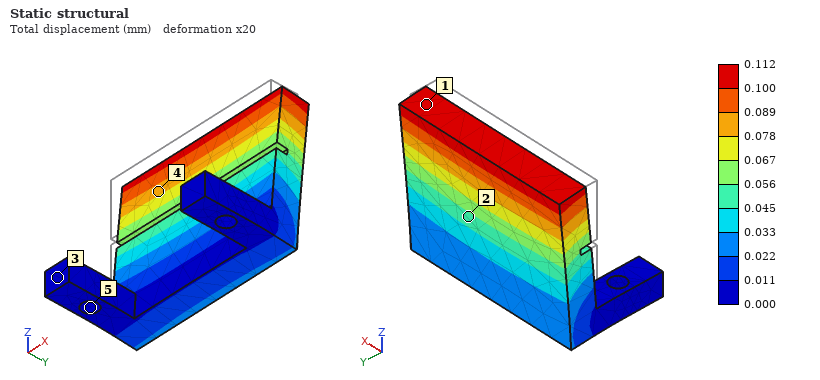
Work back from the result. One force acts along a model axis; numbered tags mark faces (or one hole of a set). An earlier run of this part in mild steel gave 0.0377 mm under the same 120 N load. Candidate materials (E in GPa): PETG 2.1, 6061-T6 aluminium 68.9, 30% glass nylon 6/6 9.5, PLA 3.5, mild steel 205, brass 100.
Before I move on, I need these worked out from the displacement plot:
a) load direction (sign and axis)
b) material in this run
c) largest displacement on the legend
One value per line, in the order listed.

+Y
6061-T6 aluminium
0.112 mm
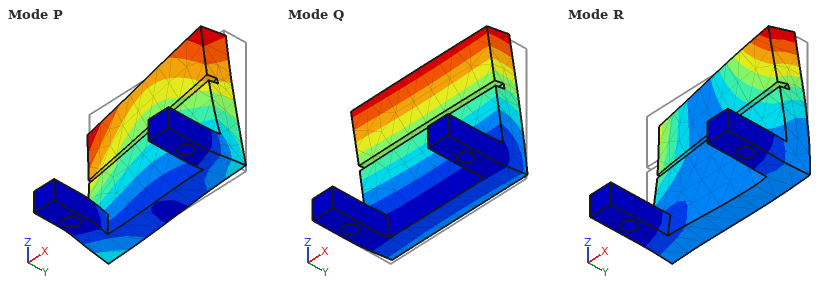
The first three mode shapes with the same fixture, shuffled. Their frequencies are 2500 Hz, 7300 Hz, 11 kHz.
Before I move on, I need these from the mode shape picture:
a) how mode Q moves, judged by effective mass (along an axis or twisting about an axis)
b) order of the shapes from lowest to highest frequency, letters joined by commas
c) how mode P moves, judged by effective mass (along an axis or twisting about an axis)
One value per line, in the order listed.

along Y
Q, P, R
along X
